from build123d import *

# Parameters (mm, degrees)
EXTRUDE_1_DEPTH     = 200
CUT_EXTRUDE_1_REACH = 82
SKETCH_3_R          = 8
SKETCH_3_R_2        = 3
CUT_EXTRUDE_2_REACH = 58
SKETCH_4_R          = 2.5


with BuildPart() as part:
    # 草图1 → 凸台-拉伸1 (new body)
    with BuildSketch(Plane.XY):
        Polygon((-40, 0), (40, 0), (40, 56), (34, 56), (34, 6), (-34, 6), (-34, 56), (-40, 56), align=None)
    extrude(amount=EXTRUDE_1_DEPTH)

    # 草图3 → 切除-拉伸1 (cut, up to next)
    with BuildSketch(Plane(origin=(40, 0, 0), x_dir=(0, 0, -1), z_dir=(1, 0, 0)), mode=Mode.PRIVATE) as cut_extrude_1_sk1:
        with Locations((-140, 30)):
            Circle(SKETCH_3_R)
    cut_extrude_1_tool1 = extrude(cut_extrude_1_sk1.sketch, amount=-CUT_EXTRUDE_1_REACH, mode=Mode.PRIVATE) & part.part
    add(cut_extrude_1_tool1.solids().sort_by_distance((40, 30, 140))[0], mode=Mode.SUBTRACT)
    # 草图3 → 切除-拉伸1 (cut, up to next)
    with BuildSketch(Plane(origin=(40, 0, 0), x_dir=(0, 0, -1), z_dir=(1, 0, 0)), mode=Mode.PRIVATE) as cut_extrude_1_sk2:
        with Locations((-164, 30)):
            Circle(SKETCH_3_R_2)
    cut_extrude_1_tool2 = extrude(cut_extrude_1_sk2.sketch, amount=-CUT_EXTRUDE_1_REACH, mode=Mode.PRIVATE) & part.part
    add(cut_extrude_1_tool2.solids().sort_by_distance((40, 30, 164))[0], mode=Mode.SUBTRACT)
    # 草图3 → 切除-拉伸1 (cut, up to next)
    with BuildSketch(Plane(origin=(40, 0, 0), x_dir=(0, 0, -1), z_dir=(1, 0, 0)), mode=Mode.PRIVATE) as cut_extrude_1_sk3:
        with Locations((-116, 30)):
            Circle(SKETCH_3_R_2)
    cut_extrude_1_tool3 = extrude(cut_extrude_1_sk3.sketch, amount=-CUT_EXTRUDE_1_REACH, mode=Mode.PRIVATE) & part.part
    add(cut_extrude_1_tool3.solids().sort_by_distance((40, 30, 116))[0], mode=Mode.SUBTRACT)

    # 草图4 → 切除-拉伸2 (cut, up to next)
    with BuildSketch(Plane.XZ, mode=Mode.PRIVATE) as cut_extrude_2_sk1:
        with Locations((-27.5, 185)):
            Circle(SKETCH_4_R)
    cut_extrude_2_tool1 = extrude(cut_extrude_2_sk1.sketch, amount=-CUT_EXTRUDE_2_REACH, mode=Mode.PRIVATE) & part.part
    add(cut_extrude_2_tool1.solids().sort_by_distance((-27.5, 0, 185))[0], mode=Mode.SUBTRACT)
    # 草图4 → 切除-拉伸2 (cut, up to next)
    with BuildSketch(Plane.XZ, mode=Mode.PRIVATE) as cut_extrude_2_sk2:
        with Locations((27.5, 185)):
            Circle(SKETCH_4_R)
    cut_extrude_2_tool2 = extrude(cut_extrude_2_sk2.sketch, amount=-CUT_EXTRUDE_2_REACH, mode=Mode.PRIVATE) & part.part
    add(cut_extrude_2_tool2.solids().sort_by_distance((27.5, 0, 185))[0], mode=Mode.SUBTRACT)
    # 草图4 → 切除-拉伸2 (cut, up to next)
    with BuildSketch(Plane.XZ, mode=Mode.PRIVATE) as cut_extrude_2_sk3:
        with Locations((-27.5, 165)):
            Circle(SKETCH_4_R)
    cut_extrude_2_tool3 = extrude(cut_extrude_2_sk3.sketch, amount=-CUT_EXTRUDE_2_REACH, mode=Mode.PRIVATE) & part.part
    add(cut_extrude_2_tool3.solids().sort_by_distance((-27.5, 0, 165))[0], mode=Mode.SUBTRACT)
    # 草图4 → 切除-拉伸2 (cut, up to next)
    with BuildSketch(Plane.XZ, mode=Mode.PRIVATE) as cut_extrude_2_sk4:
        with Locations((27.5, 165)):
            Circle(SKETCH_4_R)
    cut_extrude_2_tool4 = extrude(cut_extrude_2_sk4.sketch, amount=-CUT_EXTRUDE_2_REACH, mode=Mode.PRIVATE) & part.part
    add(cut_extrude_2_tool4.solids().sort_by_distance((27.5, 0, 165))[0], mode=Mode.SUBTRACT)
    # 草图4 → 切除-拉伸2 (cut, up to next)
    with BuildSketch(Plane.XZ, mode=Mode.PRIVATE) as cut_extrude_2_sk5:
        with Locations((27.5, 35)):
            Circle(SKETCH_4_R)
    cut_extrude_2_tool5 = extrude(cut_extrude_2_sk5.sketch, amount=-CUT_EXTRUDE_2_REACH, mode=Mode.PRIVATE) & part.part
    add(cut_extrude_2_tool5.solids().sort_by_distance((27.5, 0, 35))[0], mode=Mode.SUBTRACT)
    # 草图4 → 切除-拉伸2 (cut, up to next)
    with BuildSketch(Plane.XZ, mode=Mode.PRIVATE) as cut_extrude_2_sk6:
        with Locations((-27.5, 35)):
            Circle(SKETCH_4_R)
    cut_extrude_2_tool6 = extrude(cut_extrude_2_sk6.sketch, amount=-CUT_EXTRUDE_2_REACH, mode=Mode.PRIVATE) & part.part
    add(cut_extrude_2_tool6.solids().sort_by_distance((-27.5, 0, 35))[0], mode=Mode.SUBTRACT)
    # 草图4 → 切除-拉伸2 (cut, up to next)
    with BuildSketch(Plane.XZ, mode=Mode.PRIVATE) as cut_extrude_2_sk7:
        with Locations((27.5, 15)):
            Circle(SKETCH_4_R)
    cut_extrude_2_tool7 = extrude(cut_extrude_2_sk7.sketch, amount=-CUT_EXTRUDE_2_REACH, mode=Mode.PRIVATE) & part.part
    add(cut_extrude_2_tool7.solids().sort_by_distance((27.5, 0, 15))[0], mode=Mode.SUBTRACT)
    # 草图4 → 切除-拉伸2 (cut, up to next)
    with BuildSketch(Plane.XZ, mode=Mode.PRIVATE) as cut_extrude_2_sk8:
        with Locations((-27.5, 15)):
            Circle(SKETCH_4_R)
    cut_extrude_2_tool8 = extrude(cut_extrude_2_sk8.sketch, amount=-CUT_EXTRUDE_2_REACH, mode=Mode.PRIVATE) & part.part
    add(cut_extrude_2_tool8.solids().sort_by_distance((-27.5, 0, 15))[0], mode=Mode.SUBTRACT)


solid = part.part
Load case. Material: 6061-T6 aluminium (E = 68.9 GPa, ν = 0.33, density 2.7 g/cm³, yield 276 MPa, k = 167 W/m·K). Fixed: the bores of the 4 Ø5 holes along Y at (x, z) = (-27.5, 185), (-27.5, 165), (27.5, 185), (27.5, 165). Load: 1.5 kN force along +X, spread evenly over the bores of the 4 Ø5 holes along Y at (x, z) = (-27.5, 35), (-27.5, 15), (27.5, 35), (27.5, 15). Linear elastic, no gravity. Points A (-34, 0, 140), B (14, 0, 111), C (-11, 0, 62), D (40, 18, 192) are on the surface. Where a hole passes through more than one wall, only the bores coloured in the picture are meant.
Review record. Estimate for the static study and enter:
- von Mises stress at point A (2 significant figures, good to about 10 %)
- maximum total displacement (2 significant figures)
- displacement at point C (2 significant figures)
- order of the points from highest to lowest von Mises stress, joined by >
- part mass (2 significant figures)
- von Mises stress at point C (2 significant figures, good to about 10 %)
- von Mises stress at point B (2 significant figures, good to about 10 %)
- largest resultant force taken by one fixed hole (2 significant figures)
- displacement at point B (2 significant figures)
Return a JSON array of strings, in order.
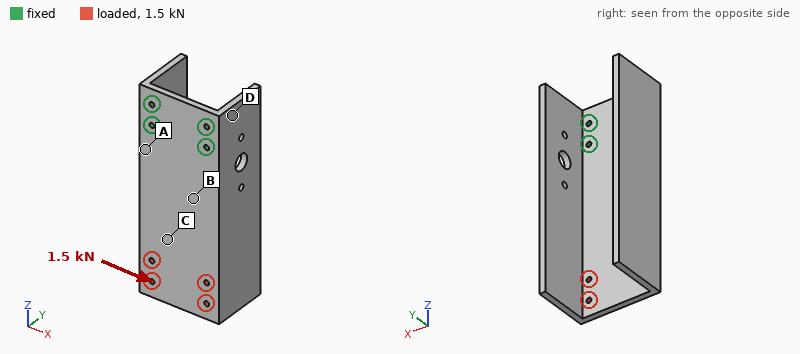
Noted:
["14 MPa", "0.13 mm", "0.050 mm", "A > B > C > D", "580 g", "4.4 MPa", "7.0 MPa", "2.7 kN", "0.022 mm"]
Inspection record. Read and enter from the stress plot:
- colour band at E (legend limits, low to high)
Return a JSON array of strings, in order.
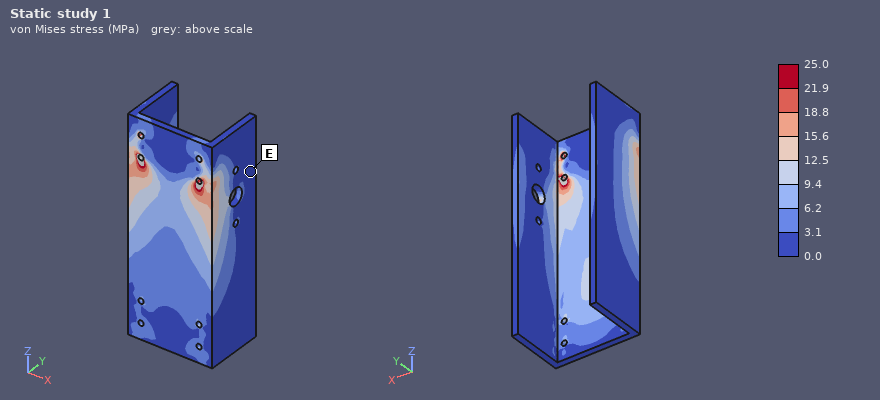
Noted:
["0.0 to 3.1 MPa"]
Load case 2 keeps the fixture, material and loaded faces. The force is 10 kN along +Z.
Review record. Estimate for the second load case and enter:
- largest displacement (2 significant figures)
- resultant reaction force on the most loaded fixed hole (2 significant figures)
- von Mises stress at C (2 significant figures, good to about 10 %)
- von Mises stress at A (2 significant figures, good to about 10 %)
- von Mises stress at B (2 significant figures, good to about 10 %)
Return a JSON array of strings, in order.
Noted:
["0.10 mm", "3.5 kN", "17 MPa", "19 MPa", "18 MPa"]
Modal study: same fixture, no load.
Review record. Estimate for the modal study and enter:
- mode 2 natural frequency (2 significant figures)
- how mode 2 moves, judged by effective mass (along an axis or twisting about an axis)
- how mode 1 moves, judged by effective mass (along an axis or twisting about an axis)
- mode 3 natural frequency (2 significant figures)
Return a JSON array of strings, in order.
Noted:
["570 Hz", "along X", "along Y", "1000 Hz"]
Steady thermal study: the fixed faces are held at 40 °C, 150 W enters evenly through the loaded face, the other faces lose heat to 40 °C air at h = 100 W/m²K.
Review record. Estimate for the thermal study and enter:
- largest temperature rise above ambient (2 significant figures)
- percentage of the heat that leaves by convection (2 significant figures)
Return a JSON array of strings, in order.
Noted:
["56 K", "86 %"]
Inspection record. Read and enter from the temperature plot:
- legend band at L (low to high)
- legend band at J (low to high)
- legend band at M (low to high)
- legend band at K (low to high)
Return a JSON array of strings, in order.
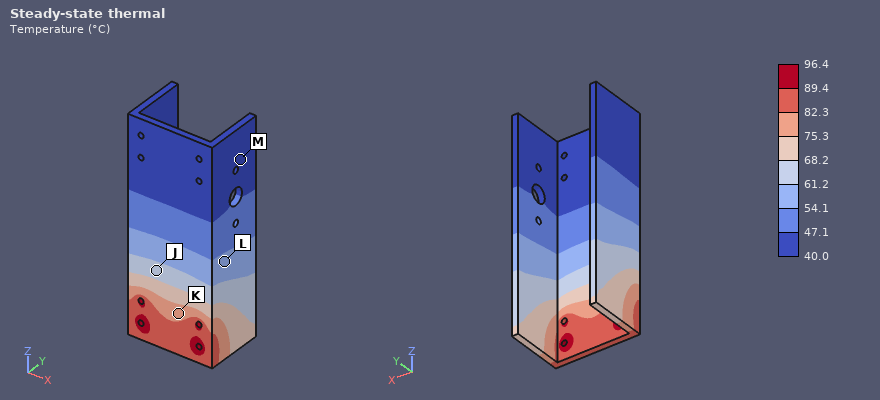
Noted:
["54.1 to 61.2 °C", "61.2 to 68.2 °C", "40.0 to 47.1 °C", "75.3 to 82.3 °C"]
